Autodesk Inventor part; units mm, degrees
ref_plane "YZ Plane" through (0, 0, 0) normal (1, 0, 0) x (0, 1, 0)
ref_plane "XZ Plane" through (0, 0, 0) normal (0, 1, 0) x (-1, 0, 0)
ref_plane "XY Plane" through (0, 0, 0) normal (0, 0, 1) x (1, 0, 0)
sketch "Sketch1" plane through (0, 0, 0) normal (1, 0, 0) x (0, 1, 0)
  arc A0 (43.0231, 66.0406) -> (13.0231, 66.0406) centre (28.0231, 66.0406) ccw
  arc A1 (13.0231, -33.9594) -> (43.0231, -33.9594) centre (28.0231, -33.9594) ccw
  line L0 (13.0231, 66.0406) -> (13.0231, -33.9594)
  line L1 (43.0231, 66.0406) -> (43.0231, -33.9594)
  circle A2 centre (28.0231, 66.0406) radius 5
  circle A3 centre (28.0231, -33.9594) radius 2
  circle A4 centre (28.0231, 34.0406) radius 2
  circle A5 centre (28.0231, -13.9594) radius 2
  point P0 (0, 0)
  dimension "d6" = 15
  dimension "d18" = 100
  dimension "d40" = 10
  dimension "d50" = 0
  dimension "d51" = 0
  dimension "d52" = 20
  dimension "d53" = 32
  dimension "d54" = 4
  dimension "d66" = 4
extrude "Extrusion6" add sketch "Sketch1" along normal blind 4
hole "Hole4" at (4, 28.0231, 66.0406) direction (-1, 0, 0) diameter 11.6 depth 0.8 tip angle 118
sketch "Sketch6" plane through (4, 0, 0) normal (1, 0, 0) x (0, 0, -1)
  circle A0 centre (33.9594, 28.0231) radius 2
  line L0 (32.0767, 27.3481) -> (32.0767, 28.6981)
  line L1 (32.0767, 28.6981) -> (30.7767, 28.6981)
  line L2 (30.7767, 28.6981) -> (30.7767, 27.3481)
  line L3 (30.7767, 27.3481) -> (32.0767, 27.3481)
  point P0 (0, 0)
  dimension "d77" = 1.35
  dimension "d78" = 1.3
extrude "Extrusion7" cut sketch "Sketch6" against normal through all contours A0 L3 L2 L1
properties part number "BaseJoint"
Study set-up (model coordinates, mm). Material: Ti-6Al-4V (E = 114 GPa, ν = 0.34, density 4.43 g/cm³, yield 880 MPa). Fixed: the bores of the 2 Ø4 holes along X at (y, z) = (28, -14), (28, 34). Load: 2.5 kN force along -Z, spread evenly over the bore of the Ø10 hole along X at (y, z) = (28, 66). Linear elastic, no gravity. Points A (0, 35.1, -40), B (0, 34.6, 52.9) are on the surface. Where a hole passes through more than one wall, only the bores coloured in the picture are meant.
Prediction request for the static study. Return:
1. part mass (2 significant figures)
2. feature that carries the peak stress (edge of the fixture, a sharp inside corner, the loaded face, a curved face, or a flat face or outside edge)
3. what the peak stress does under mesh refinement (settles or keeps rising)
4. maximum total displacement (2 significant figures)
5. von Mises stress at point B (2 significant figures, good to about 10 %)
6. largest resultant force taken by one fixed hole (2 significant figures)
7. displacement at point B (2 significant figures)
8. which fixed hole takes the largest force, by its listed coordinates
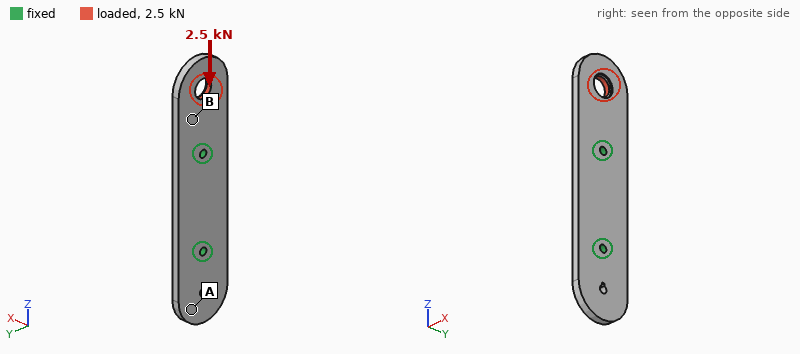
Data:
63 g
edge of the fixture
keeps rising
93 µm
42 MPa
2.1 kN
19 µm
(28, 34)
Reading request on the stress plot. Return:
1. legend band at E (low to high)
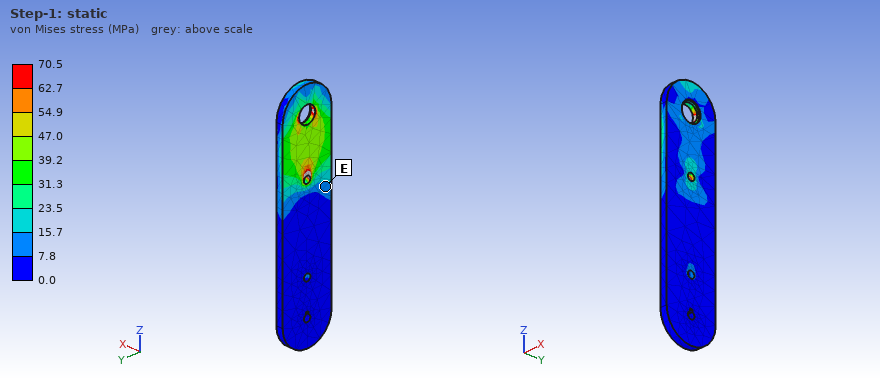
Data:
7.8 to 15.7 MPa
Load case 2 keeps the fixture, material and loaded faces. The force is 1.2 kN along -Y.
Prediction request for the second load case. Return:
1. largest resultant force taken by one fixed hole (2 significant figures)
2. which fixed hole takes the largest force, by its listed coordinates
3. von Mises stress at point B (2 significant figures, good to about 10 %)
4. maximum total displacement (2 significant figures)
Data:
1.9 kN
(28, 34)
28 MPa
68 µm
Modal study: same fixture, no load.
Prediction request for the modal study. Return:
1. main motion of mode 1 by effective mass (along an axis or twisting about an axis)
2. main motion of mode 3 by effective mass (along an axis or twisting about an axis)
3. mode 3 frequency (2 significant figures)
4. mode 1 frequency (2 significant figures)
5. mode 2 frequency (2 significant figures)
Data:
along X
twisting about Z
4700 Hz
1700 Hz
3000 Hz
